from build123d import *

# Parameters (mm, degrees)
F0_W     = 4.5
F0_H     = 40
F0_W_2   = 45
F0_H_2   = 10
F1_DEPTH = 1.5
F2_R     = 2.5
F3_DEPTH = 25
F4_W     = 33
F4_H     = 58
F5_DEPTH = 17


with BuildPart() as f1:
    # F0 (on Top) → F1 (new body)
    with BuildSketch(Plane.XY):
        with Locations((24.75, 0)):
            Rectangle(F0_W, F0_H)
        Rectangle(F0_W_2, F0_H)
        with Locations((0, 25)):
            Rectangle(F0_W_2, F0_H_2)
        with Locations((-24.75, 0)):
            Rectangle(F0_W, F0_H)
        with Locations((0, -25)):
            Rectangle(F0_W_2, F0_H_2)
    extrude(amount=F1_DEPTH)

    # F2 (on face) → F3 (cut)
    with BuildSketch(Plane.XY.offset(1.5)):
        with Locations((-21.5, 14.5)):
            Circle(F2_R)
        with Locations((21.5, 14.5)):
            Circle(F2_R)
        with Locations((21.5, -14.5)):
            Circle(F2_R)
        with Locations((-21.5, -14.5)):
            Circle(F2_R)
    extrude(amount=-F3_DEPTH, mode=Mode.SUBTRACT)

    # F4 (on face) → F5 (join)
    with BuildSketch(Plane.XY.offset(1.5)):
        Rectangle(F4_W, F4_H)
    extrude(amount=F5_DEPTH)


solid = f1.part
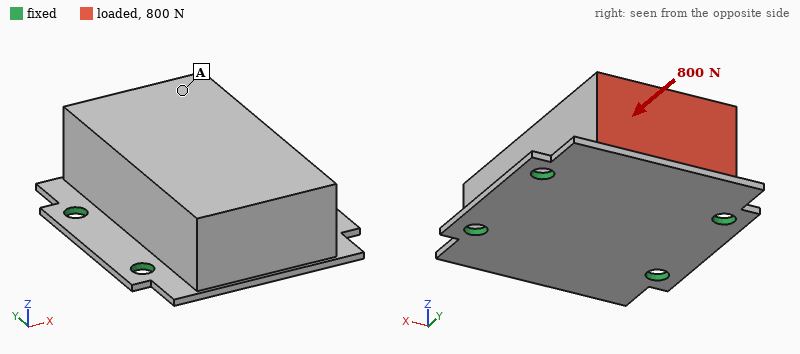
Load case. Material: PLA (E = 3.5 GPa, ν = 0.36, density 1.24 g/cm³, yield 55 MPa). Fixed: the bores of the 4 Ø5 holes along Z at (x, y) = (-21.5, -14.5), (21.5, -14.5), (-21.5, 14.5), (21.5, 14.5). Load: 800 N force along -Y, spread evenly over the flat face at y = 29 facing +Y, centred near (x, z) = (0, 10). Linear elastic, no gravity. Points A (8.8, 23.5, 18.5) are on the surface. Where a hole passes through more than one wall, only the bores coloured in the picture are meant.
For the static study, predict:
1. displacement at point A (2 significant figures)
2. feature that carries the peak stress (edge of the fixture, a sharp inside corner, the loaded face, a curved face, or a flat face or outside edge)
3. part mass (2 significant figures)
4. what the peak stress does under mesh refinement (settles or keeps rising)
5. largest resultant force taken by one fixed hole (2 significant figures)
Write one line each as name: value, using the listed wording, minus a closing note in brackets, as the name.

displacement at point A: 0.20 mm
feature that carries the peak stress: edge of the fixture
part mass: 46 g
what the peak stress does under mesh refinement: keeps rising
largest resultant force taken by one fixed hole: 250 N
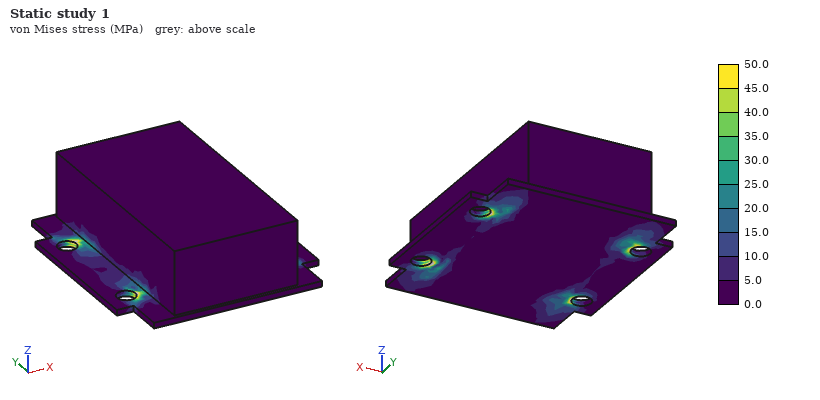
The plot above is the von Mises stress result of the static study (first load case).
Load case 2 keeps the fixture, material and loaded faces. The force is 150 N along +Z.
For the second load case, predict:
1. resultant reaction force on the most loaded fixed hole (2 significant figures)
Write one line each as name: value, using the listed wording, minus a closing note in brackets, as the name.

resultant reaction force on the most loaded fixed hole: 130 N
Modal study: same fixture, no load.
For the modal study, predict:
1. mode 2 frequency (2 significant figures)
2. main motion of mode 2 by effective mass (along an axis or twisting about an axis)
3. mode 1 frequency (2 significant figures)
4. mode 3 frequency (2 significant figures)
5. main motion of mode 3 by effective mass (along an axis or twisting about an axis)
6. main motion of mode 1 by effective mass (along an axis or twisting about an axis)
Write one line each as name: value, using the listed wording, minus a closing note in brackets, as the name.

mode 2 frequency: 1900 Hz
main motion of mode 2 by effective mass: along Z
mode 1 frequency: 1400 Hz
mode 3 frequency: 2400 Hz
main motion of mode 3 by effective mass: along X
main motion of mode 1 by effective mass: along Y
